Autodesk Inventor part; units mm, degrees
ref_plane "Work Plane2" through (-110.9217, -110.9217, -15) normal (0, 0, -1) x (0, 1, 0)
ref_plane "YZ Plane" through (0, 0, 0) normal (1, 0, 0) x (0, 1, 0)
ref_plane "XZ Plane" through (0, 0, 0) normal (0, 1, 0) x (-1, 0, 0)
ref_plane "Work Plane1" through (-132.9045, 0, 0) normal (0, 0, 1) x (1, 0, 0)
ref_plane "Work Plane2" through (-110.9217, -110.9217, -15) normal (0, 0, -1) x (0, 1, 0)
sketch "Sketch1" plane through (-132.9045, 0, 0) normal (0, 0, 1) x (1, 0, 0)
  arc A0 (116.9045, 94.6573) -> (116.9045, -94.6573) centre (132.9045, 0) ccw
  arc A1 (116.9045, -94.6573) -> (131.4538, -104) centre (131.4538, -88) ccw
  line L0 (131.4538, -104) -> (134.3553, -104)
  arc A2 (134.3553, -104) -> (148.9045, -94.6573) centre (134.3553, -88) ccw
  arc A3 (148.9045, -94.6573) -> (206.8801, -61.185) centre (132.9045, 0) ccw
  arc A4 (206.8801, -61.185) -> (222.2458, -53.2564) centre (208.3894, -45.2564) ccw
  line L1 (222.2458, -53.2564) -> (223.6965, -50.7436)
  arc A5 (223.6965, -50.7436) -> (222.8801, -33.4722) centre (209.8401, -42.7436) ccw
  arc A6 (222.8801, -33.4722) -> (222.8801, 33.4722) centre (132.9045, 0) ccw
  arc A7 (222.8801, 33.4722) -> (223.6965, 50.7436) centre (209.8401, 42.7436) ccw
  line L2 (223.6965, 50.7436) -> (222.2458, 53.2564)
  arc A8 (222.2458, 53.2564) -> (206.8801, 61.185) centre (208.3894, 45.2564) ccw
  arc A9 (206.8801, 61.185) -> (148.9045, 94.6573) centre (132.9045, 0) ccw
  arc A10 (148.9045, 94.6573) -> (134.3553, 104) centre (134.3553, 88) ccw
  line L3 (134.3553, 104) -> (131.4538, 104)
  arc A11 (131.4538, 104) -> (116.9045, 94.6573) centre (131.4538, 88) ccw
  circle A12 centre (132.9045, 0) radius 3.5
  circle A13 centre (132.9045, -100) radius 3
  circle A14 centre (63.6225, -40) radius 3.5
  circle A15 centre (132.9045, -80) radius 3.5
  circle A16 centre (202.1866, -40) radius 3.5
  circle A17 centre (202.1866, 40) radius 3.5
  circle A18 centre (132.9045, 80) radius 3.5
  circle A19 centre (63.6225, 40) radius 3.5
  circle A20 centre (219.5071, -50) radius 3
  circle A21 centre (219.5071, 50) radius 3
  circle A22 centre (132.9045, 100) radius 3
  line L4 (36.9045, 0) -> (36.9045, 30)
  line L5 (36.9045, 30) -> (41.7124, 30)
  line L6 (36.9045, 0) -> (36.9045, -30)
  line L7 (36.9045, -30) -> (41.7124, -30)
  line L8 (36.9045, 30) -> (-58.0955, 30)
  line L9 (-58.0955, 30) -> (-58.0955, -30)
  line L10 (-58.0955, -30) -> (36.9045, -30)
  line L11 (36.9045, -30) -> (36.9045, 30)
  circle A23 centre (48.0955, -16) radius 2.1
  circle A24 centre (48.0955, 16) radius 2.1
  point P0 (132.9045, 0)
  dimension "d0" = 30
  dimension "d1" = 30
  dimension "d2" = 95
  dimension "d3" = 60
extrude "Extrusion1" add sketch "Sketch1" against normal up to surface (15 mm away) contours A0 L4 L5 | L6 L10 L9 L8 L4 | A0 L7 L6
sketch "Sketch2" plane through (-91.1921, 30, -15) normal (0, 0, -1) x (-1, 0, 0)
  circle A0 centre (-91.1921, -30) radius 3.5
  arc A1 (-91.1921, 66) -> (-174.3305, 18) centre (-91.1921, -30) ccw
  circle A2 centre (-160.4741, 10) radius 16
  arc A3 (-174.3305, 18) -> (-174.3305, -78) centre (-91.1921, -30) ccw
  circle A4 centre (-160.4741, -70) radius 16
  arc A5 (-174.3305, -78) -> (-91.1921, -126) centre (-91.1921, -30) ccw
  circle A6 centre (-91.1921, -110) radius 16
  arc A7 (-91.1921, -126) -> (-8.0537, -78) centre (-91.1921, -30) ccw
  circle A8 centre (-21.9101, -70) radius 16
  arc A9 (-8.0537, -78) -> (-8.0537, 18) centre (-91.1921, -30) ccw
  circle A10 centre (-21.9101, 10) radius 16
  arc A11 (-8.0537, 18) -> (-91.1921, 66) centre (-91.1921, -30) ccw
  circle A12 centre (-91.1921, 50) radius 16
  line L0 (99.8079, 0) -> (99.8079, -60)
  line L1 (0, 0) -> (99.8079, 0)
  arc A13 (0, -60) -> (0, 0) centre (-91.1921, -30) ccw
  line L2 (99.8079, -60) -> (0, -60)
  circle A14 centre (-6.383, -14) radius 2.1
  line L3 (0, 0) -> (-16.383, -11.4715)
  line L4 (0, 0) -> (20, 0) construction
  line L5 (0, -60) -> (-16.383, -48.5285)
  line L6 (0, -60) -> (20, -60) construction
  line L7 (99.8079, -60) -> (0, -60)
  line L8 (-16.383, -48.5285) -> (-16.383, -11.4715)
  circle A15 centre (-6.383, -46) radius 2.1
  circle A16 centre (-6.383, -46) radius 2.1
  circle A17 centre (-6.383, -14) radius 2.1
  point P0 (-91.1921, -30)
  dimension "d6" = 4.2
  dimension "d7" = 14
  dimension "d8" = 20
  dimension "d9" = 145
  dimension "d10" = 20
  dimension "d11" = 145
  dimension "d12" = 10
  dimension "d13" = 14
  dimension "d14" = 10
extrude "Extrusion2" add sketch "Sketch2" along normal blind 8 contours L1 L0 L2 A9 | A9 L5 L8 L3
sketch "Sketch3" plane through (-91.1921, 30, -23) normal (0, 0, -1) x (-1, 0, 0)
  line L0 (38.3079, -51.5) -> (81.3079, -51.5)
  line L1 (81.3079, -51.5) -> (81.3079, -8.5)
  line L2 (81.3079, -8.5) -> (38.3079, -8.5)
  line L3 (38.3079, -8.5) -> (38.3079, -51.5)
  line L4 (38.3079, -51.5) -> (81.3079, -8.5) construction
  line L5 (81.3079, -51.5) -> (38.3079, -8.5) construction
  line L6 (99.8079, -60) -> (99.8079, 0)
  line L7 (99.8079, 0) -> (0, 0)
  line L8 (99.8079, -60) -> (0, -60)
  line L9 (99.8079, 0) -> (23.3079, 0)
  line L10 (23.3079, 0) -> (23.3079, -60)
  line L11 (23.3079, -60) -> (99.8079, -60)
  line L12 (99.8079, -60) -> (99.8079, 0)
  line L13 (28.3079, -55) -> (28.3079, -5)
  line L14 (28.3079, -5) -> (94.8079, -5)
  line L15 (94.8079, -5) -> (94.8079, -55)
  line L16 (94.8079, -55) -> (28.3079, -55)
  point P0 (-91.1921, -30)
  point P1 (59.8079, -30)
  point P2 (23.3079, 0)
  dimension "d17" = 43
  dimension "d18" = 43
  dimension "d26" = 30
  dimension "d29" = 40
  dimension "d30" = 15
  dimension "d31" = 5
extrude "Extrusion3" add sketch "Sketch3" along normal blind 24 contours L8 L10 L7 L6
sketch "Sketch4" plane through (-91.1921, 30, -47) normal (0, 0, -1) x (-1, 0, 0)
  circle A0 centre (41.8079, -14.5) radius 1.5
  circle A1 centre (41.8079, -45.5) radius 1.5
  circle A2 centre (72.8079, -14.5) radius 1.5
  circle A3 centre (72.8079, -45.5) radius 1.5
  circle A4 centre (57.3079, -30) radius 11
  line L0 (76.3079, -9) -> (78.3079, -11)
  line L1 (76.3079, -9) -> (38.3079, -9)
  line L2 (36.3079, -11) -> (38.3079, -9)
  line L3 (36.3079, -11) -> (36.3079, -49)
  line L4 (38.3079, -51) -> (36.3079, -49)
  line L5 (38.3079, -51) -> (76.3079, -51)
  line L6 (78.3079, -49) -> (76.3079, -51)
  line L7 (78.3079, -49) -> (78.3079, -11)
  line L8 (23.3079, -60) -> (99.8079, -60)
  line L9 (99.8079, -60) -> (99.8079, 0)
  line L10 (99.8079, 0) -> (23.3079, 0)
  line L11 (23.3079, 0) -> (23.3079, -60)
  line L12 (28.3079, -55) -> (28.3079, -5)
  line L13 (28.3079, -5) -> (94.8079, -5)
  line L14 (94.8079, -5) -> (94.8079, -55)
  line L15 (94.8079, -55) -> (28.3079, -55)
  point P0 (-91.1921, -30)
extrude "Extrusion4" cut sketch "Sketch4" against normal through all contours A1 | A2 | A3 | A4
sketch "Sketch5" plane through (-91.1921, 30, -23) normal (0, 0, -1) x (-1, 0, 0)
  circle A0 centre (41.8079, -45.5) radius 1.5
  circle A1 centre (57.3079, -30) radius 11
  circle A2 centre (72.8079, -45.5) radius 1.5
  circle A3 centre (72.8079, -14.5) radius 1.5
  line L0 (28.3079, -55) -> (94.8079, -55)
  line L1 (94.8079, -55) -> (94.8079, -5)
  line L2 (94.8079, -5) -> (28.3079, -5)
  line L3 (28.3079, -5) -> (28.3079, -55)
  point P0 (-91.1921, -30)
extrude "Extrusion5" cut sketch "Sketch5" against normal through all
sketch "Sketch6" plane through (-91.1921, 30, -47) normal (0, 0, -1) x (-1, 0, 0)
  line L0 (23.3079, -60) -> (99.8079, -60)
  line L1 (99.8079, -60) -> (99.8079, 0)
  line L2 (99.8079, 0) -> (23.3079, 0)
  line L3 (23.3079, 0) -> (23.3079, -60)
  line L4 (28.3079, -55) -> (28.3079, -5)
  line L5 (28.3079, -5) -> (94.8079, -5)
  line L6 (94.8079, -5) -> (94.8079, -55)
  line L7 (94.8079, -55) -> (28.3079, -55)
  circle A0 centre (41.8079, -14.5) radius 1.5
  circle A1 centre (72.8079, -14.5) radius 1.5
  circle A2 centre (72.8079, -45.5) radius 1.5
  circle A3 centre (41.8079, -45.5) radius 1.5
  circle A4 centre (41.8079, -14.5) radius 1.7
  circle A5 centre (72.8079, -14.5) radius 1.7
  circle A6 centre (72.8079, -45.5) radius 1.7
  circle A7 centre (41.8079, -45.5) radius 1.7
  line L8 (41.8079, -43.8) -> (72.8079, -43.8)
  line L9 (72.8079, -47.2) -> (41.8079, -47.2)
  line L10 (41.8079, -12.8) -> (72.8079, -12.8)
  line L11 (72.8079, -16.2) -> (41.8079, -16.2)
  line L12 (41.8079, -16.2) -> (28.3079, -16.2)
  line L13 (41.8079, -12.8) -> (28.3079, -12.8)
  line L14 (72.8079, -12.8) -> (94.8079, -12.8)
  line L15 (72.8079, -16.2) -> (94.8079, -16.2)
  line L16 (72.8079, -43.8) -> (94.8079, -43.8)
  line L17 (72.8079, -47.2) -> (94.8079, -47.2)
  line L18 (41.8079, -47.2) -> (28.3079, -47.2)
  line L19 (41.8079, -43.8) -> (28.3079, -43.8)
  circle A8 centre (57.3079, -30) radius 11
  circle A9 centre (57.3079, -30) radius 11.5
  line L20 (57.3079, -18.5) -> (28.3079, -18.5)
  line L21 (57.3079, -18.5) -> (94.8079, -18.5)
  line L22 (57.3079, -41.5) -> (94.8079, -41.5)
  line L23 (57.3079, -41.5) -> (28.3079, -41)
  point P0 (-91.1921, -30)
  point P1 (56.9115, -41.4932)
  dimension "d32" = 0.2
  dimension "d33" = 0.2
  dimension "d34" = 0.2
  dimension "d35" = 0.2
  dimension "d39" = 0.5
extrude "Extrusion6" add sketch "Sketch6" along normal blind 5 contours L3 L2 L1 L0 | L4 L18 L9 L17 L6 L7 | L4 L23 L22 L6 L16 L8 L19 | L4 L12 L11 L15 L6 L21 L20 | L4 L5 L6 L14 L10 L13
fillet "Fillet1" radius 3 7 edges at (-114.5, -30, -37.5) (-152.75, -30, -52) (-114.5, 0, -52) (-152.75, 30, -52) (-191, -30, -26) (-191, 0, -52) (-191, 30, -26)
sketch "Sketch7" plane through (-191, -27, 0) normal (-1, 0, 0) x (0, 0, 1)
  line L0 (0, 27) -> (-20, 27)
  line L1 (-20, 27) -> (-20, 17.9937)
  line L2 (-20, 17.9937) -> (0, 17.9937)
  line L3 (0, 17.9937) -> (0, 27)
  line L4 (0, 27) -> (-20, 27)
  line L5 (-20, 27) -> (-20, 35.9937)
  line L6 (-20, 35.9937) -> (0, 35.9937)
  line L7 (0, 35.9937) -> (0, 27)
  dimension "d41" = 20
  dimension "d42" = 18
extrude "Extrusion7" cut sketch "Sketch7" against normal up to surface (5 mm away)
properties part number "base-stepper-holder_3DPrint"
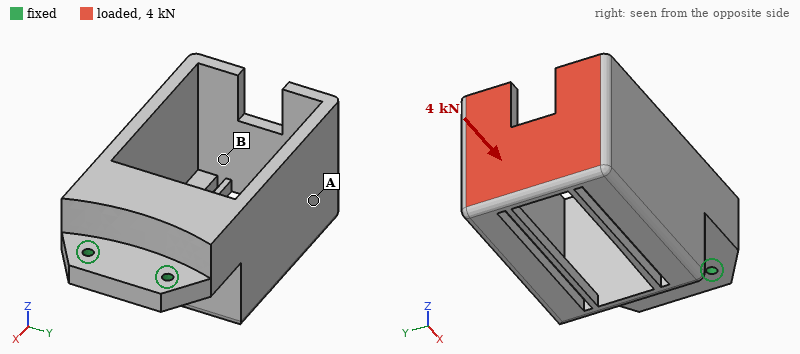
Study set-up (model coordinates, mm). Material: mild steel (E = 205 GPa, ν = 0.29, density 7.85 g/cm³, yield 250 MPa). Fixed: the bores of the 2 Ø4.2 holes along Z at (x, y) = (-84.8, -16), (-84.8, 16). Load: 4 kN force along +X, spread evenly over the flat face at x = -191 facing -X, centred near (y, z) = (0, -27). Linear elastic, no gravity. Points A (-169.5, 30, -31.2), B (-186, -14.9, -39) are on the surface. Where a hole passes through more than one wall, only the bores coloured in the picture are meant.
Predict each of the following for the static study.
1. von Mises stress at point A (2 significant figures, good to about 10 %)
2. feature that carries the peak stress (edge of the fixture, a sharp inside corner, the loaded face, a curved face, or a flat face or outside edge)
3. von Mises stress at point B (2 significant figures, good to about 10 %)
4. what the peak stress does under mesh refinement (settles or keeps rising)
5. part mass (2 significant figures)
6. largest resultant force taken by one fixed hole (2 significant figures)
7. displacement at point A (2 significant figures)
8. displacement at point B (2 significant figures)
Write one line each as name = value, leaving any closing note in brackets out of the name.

von Mises stress at point A = 11 MPa
feature that carries the peak stress = edge of the fixture
von Mises stress at point B = 27 MPa
what the peak stress does under mesh refinement = keeps rising
part mass = 830 g
largest resultant force taken by one fixed hole = 2.0 kN
displacement at point A = 0.11 mm
displacement at point B = 0.13 mm
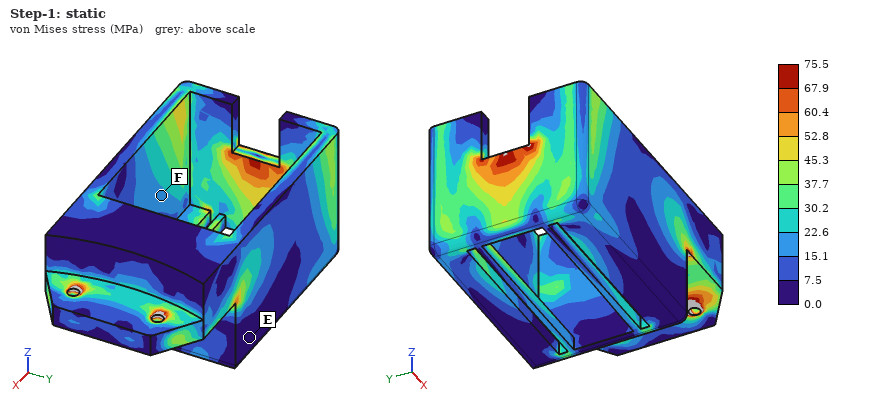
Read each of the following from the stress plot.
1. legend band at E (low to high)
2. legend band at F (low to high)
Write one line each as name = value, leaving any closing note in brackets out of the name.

legend band at E = 0.0 to 7.5 MPa
legend band at F = 15.1 to 22.6 MPa
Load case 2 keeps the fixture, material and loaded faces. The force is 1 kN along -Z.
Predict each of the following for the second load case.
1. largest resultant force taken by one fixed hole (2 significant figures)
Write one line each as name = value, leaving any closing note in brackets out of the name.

largest resultant force taken by one fixed hole = 510 N
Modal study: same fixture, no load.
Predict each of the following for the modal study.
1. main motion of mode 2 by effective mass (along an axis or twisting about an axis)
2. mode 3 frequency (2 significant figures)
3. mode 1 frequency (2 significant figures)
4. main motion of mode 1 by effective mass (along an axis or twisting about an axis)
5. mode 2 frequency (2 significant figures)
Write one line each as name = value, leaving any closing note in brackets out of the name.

main motion of mode 2 by effective mass = along Y
mode 3 frequency = 1700 Hz
mode 1 frequency = 500 Hz
main motion of mode 1 by effective mass = along Z
mode 2 frequency = 850 Hz
